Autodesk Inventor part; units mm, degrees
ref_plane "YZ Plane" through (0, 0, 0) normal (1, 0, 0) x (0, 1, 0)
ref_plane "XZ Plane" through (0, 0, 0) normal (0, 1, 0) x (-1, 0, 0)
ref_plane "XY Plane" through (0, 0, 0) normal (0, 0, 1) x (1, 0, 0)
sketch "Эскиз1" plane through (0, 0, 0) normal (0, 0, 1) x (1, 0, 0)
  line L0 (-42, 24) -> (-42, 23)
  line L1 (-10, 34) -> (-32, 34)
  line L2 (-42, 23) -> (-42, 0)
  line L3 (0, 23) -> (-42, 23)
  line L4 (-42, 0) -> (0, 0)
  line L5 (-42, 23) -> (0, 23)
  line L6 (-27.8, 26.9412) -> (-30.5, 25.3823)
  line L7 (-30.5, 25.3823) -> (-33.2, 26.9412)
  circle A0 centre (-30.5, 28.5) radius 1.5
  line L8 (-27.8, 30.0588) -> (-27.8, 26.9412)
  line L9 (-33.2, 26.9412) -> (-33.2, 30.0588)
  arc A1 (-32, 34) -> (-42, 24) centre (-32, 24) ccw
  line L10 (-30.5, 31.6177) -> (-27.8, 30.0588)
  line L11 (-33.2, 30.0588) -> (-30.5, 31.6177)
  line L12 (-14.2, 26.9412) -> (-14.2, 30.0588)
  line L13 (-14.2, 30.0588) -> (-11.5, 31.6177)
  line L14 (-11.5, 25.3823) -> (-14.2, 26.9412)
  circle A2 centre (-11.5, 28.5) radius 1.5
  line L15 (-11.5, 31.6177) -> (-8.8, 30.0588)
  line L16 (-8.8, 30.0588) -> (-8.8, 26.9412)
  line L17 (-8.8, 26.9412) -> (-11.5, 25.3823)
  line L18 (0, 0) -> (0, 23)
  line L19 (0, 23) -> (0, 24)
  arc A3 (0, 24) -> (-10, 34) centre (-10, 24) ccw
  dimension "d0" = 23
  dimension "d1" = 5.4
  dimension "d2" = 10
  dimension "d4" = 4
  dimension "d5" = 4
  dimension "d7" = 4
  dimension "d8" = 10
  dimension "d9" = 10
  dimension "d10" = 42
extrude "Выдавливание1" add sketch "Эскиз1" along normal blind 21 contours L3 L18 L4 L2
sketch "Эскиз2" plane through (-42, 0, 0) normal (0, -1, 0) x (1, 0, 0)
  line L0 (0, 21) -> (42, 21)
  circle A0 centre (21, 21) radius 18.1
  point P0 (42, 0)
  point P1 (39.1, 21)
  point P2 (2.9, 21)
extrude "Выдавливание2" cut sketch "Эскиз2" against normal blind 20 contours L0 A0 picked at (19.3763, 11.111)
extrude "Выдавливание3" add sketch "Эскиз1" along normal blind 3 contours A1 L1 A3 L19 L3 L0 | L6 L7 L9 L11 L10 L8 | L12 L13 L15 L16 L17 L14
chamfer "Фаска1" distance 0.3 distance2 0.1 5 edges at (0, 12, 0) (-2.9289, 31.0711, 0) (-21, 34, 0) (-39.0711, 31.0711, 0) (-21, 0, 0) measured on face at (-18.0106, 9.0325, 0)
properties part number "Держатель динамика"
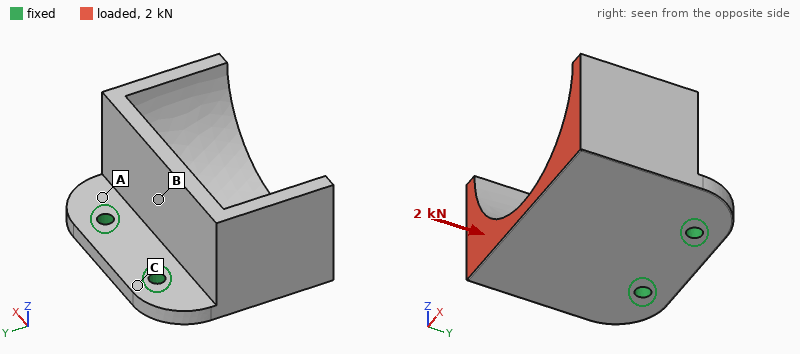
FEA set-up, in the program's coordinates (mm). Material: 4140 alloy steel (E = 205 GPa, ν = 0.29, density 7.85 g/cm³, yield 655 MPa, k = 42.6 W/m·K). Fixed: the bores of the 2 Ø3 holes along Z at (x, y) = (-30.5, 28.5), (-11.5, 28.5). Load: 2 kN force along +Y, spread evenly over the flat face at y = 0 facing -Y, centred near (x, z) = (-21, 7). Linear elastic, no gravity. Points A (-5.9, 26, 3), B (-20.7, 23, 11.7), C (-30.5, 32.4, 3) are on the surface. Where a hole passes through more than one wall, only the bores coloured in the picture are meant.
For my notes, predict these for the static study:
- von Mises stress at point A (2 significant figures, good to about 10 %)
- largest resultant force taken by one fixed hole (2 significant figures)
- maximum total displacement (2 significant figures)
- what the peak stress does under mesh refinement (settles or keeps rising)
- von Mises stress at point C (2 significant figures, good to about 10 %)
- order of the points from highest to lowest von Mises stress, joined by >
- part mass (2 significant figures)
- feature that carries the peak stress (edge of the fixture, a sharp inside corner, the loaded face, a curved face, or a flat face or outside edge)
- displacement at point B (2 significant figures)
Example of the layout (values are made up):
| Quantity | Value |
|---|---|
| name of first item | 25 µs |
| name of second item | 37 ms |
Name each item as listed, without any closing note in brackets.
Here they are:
| Quantity | Value |
|---|---|
| von Mises stress at point A | 140 MPa |
| largest resultant force taken by one fixed hole | 1.0 kN |
| maximum total displacement | 0.14 mm |
| what the peak stress does under mesh refinement | keeps rising |
| von Mises stress at point C | 48 MPa |
| order of the points from highest to lowest von Mises stress, joined by > | A > C > B |
| part mass | 88 g |
| feature that carries the peak stress | edge of the fixture |
| displacement at point B | 0.045 mm |
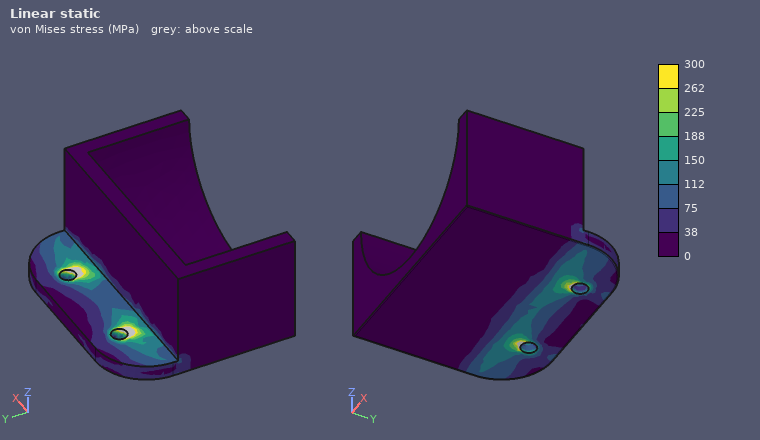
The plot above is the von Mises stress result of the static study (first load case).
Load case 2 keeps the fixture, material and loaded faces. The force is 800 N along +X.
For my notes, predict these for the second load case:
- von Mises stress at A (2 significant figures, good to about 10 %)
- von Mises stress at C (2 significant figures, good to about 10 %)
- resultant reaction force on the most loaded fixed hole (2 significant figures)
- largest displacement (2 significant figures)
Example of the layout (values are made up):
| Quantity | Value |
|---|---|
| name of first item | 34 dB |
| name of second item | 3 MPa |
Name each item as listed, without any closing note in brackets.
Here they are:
| Quantity | Value |
|---|---|
| von Mises stress at A | 14 MPa |
| von Mises stress at C | 18 MPa |
| resultant reaction force on the most loaded fixed hole | 1.2 kN |
| largest displacement | 16 µm |
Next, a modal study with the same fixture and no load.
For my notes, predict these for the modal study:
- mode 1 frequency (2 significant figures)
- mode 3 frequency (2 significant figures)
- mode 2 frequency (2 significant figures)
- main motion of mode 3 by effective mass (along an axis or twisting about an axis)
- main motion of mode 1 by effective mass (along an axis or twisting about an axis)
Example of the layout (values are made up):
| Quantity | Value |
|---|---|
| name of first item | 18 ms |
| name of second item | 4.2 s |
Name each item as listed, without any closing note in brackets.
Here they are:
| Quantity | Value |
|---|---|
| mode 1 frequency | 1700 Hz |
| mode 3 frequency | 7700 Hz |
| mode 2 frequency | 3800 Hz |
| main motion of mode 3 by effective mass | along X |
| main motion of mode 1 by effective mass | along Z |
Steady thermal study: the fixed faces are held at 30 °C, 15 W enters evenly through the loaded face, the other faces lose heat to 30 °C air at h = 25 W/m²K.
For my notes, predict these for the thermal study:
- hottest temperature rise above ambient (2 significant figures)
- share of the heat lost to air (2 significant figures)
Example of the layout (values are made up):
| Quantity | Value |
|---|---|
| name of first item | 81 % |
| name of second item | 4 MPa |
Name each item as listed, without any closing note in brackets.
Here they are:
| Quantity | Value |
|---|---|
| hottest temperature rise above ambient | 43 K |
| share of the heat lost to air | 24 % |
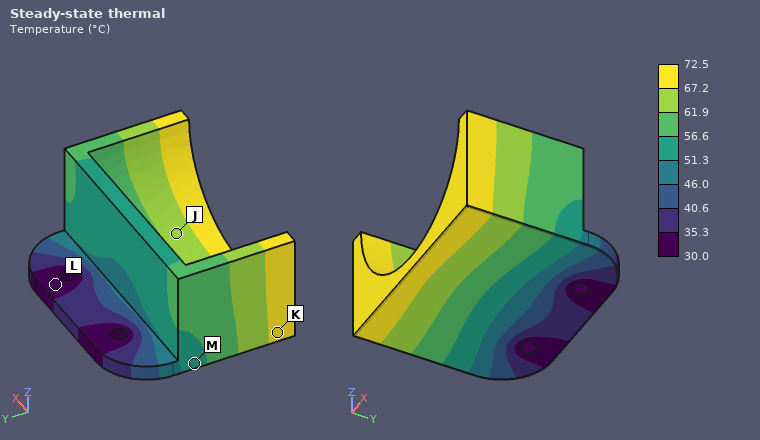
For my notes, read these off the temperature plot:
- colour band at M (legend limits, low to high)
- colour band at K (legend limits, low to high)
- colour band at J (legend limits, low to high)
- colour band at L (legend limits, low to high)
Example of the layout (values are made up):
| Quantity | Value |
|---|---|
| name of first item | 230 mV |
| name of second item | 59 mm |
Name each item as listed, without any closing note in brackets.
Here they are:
| Quantity | Value |
|---|---|
| colour band at M | 51.3 to 56.6 °C |
| colour band at K | 67.2 to 72.5 °C |
| colour band at J | 61.9 to 67.2 °C |
| colour band at L | 30.0 to 35.3 °C |
